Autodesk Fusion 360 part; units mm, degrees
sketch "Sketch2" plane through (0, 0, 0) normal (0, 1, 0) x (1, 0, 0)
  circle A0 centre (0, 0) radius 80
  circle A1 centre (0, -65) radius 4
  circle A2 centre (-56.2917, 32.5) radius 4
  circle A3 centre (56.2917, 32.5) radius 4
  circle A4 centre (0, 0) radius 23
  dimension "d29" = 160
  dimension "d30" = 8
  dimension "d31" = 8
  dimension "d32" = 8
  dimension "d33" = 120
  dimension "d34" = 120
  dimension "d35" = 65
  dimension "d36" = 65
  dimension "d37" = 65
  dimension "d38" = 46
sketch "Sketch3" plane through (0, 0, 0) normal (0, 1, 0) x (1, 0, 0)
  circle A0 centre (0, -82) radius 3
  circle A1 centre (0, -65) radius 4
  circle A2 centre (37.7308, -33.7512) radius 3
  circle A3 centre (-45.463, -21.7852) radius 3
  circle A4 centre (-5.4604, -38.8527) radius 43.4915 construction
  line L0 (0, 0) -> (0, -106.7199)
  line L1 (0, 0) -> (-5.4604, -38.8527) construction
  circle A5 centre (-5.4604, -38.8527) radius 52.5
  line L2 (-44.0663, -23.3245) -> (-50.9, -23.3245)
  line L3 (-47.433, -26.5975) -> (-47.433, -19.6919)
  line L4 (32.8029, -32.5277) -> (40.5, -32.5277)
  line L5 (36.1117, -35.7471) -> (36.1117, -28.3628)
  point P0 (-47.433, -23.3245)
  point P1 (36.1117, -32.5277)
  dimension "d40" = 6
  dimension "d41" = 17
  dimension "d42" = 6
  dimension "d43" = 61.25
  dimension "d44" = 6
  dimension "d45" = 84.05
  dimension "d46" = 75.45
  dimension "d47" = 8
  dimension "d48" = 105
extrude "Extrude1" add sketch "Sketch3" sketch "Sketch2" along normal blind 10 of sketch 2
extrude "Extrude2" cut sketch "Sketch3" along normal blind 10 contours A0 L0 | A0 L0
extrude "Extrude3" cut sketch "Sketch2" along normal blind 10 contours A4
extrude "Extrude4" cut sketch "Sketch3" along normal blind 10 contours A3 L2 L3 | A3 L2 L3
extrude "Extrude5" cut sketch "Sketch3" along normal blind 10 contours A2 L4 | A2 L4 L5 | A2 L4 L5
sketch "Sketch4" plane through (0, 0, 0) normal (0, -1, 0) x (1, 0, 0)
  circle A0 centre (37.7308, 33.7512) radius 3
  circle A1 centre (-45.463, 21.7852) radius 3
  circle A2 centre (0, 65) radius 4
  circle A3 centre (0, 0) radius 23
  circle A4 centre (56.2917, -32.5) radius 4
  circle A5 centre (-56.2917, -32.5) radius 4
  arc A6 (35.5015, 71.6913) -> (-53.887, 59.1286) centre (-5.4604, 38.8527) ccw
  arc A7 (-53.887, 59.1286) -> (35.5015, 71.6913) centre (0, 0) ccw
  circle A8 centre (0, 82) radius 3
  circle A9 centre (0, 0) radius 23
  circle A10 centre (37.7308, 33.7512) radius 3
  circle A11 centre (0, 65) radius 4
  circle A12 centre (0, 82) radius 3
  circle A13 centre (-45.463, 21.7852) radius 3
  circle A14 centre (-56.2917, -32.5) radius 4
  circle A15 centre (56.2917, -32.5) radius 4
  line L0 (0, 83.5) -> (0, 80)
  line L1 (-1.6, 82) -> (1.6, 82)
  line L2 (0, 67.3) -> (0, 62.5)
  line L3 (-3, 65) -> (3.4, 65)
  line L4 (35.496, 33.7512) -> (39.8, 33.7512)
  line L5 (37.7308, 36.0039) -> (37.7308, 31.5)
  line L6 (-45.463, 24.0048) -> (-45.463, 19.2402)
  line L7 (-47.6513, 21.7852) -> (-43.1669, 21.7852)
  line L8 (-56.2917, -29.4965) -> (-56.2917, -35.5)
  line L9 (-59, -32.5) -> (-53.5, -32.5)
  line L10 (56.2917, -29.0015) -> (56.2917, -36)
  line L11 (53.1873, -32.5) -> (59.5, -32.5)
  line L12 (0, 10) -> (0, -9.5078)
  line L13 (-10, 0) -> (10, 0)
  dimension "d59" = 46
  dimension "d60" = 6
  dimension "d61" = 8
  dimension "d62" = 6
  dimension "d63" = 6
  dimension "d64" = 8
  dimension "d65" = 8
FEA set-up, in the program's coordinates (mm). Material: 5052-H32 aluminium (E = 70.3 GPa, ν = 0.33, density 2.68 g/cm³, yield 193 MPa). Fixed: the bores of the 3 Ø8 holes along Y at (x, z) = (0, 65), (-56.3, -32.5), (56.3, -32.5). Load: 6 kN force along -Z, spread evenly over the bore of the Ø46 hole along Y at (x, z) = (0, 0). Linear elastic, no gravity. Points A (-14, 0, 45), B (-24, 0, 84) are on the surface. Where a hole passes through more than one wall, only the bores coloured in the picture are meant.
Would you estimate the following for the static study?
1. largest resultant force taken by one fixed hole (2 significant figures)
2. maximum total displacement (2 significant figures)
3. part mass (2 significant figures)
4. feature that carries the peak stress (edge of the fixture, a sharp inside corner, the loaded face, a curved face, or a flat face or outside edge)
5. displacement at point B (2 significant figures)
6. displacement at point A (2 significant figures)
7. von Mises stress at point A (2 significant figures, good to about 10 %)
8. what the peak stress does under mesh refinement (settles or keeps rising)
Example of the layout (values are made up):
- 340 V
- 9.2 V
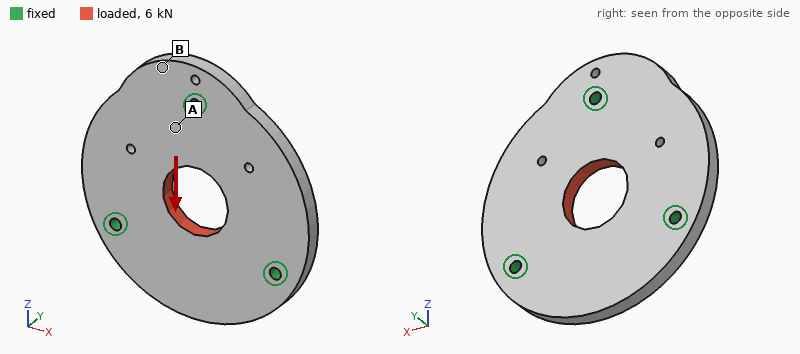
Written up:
- 2.0 kN
- 6.6 µm
- 510 g
- edge of the fixture
- 1.6 µm
- 2.2 µm
- 4.4 MPa
- keeps rising
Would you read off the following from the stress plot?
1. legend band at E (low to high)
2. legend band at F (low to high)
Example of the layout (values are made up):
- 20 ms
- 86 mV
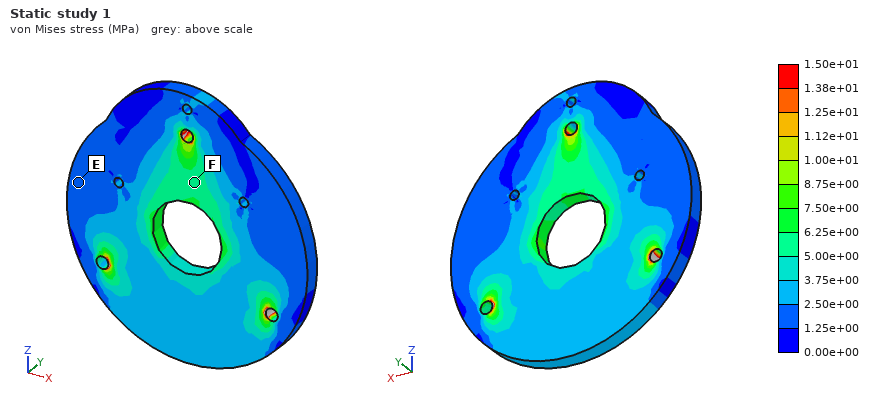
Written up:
- 1.25e+00 to 2.50e+00 MPa
- 5.00e+00 to 6.25e+00 MPa
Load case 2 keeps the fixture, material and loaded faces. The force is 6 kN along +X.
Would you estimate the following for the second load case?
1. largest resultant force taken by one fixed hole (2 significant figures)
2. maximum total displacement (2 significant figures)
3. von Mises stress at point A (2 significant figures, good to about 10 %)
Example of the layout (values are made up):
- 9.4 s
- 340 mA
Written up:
- 2.0 kN
- 6.2 µm
- 3.0 MPa
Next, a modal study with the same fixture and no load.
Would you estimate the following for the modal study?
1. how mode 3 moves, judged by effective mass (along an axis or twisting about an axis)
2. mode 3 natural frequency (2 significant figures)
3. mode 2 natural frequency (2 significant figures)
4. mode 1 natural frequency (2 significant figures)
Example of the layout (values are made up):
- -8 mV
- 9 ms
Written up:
- along Y
- 2900 Hz
- 2500 Hz
- 2500 Hz
